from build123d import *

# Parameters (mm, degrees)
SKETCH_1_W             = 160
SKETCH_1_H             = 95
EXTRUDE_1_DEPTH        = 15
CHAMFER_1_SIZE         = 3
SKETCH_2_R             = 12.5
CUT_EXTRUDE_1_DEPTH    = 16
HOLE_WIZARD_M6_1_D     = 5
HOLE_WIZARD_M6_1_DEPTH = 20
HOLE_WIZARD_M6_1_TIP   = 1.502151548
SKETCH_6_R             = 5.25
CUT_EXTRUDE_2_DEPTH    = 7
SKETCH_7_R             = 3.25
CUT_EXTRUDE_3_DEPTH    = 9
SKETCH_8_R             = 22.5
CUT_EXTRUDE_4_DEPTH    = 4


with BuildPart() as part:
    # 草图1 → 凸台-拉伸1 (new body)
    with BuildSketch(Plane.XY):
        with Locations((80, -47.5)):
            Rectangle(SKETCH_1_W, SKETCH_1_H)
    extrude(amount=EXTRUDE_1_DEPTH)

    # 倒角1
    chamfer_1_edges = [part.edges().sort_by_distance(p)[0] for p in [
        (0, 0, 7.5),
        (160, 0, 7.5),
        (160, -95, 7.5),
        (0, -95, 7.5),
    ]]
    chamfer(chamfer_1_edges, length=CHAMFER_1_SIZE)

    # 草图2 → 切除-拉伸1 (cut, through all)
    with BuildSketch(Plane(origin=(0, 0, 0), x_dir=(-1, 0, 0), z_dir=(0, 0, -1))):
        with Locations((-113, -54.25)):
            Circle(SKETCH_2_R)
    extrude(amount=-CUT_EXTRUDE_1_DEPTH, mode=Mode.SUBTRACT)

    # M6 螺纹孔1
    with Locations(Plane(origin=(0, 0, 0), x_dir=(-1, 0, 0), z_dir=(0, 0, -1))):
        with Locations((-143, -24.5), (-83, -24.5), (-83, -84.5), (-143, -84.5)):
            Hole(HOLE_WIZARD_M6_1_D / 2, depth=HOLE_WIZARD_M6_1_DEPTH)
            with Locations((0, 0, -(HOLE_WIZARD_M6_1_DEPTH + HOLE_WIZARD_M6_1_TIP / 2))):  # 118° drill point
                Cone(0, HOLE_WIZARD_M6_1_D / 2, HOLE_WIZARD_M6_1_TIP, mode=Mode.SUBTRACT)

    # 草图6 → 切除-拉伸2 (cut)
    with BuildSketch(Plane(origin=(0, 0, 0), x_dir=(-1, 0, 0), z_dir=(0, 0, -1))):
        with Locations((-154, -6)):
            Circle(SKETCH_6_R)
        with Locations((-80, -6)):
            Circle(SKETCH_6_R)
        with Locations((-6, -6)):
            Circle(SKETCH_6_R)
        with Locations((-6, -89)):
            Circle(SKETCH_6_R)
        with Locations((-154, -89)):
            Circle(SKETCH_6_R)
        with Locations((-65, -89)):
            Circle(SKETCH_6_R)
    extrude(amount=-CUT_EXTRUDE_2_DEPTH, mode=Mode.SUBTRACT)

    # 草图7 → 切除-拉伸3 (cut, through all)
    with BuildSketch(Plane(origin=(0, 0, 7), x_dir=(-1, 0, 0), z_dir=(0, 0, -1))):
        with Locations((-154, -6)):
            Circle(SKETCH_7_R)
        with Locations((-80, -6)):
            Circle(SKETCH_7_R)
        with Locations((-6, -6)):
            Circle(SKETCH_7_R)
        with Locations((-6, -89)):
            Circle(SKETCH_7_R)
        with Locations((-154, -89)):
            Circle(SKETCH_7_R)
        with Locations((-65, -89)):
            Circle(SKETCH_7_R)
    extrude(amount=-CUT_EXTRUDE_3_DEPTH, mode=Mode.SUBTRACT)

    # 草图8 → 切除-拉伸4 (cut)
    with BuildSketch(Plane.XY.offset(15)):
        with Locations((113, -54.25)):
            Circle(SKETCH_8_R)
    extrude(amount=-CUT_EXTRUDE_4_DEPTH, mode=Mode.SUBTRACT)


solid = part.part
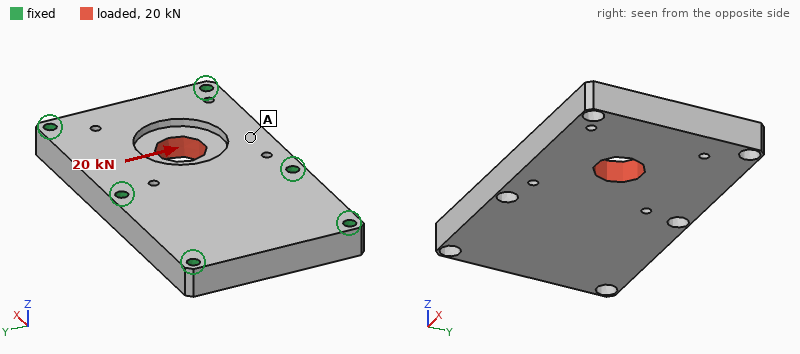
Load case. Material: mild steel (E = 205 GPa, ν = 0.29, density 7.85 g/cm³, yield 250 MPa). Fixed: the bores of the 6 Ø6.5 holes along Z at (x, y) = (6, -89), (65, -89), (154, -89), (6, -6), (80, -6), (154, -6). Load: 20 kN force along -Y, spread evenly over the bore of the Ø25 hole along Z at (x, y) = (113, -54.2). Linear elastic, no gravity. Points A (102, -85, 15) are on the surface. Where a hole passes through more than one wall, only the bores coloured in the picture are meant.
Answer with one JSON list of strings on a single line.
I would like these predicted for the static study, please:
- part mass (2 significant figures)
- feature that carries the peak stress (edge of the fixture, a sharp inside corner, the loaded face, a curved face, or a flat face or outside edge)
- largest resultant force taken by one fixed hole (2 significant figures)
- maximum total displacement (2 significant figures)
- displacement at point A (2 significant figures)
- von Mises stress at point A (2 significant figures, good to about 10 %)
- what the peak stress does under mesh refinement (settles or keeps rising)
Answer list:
["1.6 kg", "edge of the fixture", "5.7 kN", "7.7 µm", "5.4 µm", "8.7 MPa", "keeps rising"]
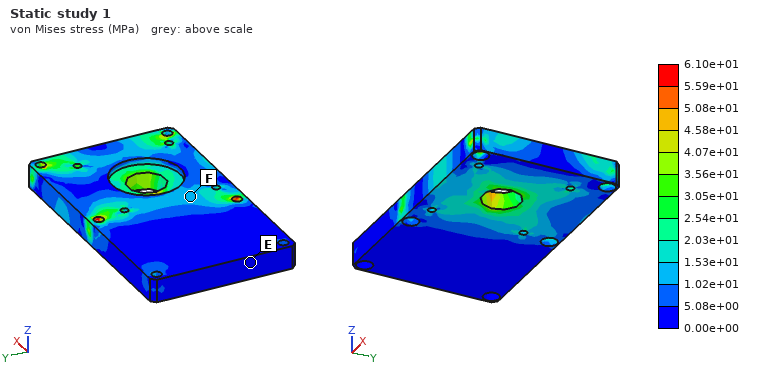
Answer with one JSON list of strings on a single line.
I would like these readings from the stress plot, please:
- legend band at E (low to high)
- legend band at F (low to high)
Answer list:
["0.00e+00 to 5.08e+00 MPa", "1.02e+01 to 1.53e+01 MPa"]
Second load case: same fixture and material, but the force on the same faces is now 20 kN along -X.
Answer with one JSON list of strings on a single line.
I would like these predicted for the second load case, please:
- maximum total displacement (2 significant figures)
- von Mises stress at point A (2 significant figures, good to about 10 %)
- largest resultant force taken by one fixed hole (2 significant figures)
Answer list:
["6.7 µm", "7.7 MPa", "5.1 kN"]
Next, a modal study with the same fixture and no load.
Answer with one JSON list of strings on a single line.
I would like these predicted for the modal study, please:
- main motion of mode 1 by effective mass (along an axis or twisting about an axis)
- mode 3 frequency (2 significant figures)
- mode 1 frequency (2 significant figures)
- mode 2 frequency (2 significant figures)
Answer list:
["along Z", "8200 Hz", "5400 Hz", "6400 Hz"]
